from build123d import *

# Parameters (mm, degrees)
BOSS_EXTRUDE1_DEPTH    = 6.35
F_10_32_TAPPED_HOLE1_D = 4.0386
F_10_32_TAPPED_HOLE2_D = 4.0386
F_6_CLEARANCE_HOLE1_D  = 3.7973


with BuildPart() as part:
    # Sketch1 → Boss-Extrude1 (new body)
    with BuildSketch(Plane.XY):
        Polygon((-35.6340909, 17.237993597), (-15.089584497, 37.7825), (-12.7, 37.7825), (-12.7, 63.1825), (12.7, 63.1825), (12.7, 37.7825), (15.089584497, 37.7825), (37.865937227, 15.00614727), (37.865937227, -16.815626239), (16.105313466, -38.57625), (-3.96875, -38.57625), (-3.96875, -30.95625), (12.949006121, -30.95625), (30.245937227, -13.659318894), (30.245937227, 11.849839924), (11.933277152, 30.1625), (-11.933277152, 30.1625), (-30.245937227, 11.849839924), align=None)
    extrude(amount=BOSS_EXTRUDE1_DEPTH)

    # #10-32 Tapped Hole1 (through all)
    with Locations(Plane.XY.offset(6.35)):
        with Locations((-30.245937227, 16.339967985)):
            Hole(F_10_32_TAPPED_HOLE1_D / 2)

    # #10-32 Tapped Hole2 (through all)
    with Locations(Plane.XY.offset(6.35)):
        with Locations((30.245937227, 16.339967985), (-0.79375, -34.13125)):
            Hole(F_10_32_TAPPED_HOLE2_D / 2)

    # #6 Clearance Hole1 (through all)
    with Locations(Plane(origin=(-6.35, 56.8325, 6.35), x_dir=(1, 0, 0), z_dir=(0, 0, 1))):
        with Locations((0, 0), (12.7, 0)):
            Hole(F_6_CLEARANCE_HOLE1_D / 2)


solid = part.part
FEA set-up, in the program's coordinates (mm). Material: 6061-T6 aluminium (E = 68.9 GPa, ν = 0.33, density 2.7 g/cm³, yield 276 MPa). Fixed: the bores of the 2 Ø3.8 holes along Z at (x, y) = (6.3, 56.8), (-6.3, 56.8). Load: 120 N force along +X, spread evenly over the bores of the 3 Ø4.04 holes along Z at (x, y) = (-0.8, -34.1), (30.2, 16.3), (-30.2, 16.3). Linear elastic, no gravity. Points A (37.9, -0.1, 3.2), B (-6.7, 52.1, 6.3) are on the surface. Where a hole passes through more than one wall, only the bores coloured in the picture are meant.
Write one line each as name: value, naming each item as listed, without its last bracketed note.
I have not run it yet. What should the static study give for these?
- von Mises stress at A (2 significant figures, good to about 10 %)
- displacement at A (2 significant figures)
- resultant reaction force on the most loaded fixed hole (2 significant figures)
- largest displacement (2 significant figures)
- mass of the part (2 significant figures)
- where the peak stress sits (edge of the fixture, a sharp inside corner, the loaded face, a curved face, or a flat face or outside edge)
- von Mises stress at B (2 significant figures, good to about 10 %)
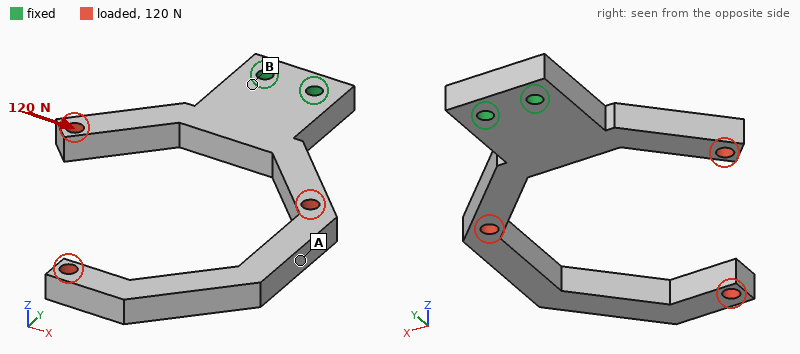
von Mises stress at A: 22 MPa
displacement at A: 0.21 mm
resultant reaction force on the most loaded fixed hole: 460 N
largest displacement: 0.57 mm
mass of the part: 31 g
where the peak stress sits: the loaded face
von Mises stress at B: 7.5 MPa
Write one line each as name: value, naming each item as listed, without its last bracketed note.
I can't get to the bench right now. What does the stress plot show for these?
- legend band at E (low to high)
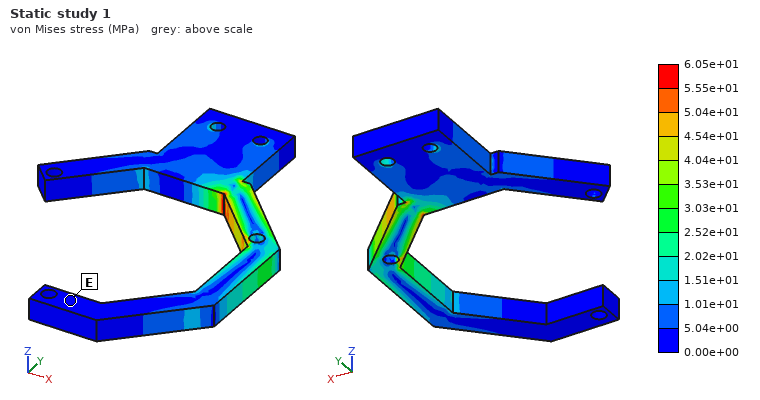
legend band at E: 0.00e+00 to 5.04e+00 MPa
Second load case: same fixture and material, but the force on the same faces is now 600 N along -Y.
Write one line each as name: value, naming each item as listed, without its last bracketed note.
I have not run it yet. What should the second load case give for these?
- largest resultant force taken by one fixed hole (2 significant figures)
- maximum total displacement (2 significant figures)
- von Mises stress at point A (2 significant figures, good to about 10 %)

largest resultant force taken by one fixed hole: 310 N
maximum total displacement: 1.4 mm
von Mises stress at point A: 110 MPa
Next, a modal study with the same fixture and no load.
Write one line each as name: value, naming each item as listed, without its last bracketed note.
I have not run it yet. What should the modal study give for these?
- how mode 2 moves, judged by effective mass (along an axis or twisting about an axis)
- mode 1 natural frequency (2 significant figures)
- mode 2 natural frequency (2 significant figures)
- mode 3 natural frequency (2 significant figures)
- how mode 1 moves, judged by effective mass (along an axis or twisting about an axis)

how mode 2 moves, judged by effective mass: along X
mode 1 natural frequency: 440 Hz
mode 2 natural frequency: 650 Hz
mode 3 natural frequency: 1400 Hz
how mode 1 moves, judged by effective mass: along Z
